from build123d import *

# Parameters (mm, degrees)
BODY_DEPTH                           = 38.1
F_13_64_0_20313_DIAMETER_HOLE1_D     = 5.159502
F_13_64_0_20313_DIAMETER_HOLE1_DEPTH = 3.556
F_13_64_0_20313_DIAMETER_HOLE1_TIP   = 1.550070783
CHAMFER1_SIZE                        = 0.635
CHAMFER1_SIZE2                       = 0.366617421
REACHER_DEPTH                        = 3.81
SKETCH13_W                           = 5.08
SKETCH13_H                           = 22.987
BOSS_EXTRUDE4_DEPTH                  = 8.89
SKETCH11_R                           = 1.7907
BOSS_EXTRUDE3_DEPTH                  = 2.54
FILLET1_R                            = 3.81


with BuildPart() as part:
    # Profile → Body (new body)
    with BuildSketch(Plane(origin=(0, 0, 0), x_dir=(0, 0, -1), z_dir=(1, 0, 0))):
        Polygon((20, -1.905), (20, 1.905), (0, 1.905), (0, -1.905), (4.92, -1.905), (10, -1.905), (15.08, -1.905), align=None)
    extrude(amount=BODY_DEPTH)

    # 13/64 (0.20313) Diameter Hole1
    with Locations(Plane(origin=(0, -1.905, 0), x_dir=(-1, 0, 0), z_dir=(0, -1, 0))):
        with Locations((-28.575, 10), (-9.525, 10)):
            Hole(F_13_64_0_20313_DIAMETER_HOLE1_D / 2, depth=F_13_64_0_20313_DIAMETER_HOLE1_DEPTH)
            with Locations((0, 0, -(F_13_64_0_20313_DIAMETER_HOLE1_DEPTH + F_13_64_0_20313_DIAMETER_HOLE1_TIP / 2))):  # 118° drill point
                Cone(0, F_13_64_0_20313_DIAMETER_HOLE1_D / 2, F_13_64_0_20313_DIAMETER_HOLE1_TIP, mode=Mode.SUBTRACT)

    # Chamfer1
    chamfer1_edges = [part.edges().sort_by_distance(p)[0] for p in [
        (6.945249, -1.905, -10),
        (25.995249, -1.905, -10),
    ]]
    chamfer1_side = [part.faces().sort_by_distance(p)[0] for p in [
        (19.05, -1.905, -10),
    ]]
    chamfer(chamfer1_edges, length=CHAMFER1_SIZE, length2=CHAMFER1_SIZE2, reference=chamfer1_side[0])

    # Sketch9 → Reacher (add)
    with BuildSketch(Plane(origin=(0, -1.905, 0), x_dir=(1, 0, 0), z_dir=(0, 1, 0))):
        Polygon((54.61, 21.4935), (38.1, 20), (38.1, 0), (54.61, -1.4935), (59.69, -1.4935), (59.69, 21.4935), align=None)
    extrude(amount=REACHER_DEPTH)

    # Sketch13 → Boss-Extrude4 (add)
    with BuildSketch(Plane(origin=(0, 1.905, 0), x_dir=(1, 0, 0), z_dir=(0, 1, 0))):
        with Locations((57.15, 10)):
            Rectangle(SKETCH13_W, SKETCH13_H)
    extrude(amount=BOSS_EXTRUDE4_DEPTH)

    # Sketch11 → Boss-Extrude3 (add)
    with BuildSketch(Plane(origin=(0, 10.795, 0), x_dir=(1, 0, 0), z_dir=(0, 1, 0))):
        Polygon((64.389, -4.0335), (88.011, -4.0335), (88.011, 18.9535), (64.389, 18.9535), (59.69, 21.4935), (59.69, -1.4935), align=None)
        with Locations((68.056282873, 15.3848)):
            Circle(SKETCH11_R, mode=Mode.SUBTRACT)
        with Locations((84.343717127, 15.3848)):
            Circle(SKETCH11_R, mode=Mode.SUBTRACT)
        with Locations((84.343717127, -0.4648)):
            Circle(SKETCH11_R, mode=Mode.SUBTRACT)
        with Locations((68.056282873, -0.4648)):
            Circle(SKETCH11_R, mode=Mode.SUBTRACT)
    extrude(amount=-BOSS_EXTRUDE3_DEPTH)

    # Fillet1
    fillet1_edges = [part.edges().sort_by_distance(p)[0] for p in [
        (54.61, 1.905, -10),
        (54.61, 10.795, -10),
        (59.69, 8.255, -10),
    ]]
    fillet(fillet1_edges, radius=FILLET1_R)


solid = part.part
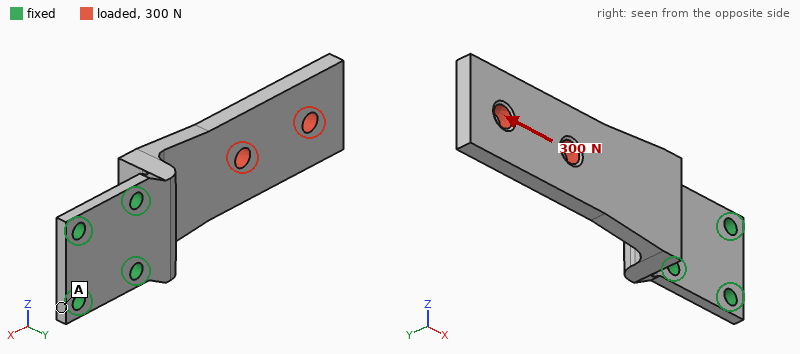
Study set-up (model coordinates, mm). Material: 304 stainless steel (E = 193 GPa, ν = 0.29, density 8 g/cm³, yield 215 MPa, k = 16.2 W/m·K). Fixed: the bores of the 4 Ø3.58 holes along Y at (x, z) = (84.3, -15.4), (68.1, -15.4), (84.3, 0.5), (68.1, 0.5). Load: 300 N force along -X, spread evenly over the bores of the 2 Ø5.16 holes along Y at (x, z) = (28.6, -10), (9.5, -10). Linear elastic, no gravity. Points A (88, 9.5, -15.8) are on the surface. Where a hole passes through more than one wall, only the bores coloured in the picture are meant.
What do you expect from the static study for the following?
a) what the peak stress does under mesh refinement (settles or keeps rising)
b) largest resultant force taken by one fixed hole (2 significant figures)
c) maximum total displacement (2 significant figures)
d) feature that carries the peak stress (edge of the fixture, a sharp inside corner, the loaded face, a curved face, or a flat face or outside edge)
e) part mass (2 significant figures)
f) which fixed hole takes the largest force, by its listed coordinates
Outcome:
keeps rising
180 N
0.21 mm
edge of the fixture
58 g
(68.1, -15.4)
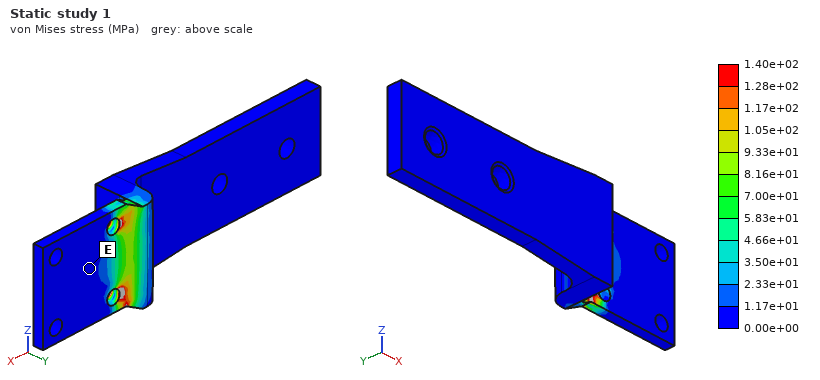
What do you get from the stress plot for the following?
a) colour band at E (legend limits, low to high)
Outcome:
0.00e+00 to 1.17e+01 MPa
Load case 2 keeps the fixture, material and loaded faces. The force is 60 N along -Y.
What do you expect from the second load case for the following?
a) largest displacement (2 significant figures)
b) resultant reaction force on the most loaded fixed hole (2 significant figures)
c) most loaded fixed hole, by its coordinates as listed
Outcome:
0.29 mm
49 N
(68.1, -15.4)
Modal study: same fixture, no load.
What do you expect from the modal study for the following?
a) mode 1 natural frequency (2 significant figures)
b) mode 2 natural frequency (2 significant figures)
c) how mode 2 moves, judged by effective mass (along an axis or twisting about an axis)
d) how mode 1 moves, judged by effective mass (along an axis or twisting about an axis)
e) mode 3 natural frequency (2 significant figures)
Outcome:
550 Hz
2400 Hz
along Z
along Y
3000 Hz
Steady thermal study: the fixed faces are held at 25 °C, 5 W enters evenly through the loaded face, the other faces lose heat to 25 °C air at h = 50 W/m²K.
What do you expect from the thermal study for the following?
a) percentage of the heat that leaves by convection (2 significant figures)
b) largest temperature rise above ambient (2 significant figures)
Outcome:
88 %
49 K
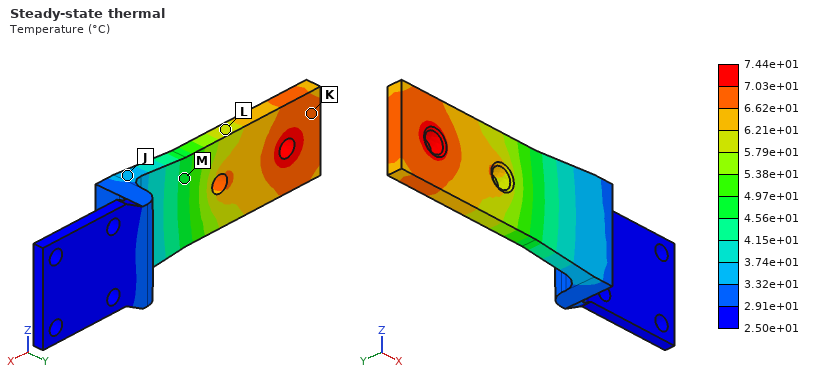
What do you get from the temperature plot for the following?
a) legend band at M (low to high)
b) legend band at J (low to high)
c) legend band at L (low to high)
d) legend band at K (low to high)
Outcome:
4.56e+01 to 4.97e+01 °C
3.32e+01 to 3.74e+01 °C
5.79e+01 to 6.21e+01 °C
6.62e+01 to 7.03e+01 °C
